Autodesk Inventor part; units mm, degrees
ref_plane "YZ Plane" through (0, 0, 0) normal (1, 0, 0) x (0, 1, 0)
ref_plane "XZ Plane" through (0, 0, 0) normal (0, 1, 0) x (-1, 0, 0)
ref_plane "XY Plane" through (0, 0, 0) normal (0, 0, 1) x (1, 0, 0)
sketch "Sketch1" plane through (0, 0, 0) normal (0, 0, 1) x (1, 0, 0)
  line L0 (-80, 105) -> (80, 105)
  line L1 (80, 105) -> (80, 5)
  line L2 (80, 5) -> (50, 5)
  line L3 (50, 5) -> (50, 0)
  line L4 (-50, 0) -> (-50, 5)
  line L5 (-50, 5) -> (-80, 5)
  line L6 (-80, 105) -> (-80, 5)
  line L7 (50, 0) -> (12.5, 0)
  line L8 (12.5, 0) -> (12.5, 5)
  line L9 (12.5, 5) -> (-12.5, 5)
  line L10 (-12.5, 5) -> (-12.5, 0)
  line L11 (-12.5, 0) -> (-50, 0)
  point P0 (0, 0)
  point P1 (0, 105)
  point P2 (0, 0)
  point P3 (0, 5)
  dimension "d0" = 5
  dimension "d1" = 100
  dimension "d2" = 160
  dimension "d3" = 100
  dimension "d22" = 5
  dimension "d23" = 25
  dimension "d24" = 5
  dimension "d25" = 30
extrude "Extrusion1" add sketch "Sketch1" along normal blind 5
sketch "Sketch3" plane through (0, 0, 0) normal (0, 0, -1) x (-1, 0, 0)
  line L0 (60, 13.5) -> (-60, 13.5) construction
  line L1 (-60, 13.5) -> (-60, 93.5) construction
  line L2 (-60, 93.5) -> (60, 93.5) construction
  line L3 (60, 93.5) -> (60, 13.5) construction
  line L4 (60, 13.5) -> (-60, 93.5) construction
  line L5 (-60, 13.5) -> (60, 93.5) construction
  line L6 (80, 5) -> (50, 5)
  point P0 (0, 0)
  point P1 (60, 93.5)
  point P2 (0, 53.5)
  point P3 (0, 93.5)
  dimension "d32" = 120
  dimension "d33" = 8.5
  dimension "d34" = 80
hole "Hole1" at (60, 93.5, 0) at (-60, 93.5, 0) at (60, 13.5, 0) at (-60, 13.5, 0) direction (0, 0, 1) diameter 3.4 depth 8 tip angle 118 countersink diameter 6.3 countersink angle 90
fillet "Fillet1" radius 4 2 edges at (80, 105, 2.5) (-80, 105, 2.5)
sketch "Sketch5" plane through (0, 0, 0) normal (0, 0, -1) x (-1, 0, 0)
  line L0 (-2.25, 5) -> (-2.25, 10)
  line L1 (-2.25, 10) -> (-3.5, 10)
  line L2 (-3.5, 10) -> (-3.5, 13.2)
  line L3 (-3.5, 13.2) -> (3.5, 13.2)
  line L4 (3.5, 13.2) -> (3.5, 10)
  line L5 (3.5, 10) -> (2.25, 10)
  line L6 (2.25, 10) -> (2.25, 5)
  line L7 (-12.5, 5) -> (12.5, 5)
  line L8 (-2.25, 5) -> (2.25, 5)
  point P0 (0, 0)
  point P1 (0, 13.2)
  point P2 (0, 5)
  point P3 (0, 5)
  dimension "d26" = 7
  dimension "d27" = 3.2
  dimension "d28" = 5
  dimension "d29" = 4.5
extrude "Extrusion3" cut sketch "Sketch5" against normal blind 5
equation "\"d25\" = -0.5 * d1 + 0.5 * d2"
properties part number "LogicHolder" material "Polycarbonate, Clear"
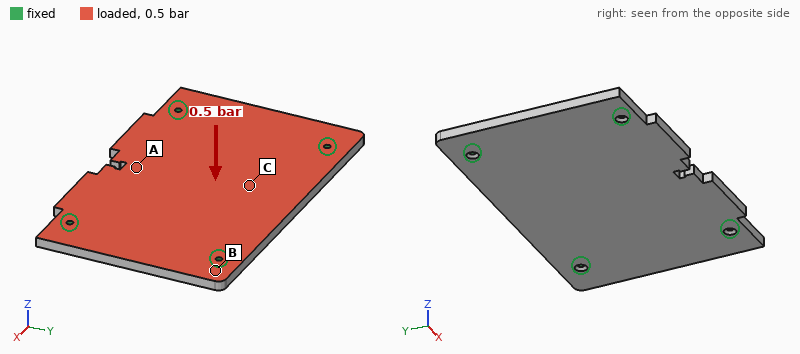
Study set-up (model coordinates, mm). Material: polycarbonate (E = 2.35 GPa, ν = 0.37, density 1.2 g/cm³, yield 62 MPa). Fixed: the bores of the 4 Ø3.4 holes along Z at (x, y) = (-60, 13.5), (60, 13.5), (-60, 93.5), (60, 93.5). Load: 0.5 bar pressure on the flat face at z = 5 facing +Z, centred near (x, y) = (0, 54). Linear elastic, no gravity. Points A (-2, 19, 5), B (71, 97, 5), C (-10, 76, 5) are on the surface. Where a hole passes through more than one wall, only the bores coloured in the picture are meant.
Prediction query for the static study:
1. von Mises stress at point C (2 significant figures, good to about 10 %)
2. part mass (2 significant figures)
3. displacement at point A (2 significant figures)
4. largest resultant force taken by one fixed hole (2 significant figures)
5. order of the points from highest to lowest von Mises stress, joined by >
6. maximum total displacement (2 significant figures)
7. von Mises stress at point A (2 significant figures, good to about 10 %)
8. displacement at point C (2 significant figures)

7.9 MPa
98 g
2.0 mm
230 N
A > C > B
2.1 mm
13 MPa
1.9 mm
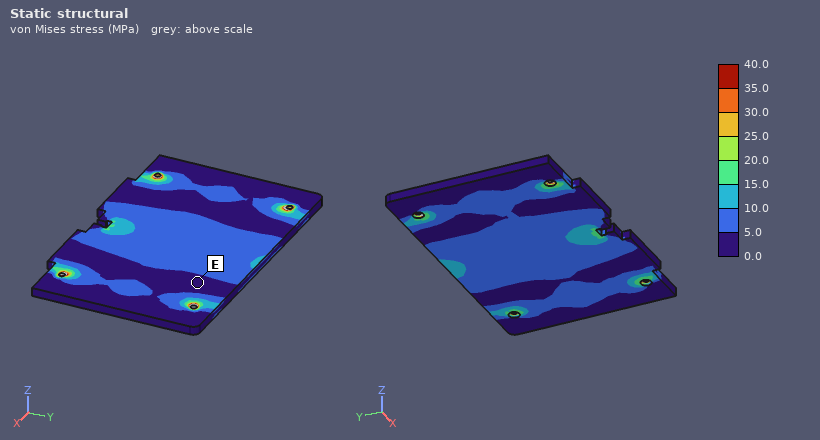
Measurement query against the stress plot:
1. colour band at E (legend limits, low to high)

0.0 to 5.0 MPa
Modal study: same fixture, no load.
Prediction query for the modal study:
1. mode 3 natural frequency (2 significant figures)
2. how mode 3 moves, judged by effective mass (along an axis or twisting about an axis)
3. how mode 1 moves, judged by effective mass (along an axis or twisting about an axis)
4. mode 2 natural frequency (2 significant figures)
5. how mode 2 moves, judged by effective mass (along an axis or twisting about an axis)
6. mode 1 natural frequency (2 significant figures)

800 Hz
along Z
along Z
560 Hz
twisting about X
360 Hz
